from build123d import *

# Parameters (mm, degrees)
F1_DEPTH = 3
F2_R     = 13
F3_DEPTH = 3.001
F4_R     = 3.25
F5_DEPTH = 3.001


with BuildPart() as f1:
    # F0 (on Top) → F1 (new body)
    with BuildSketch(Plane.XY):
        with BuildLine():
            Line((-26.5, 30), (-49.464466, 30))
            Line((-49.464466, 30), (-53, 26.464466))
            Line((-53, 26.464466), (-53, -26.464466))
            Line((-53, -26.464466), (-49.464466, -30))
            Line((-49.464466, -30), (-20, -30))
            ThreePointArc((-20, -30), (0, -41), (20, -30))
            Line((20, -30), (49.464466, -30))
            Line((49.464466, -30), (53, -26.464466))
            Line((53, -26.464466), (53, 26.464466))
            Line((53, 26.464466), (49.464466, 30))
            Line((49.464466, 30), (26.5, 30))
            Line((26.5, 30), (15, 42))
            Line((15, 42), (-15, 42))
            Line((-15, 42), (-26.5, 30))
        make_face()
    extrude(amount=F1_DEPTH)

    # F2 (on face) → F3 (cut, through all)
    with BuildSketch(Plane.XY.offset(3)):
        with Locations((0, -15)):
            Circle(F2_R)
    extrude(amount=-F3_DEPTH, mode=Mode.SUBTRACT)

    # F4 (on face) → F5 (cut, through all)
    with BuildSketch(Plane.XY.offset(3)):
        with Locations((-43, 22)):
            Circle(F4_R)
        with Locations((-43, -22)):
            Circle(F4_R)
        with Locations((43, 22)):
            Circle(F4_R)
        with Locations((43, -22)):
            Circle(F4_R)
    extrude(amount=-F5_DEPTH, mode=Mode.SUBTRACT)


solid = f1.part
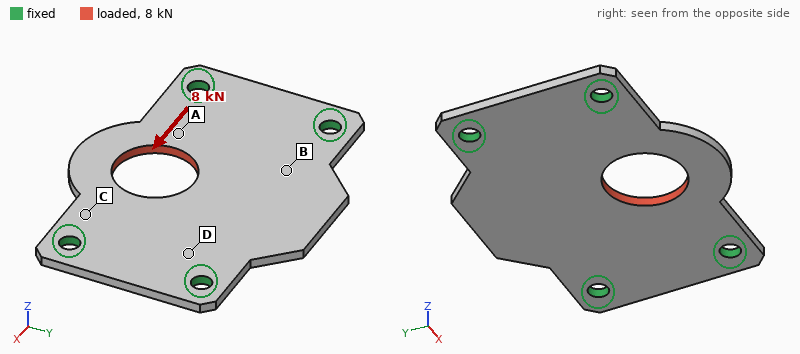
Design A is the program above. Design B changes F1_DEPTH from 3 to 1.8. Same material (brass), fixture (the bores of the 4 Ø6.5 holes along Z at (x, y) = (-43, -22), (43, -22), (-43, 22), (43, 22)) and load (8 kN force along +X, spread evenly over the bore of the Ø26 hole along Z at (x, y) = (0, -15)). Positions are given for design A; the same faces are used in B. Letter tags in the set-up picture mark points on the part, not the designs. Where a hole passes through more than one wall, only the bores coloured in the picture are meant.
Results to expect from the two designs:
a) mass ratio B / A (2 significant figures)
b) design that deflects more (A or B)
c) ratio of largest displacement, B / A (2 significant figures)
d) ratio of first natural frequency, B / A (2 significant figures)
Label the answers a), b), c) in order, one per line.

a) 0.60
b) B
c) 1.7
d) 0.61
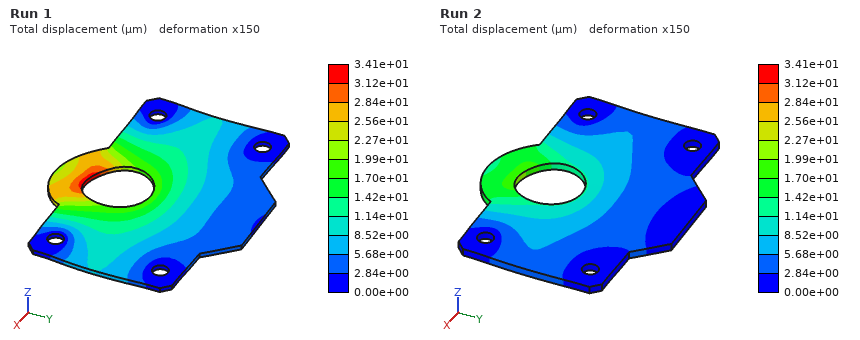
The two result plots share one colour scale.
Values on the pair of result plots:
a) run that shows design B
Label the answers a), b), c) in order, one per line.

a) Run 1
